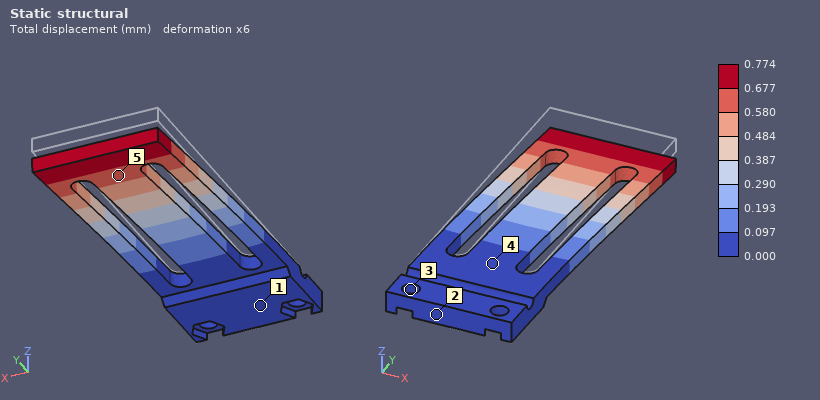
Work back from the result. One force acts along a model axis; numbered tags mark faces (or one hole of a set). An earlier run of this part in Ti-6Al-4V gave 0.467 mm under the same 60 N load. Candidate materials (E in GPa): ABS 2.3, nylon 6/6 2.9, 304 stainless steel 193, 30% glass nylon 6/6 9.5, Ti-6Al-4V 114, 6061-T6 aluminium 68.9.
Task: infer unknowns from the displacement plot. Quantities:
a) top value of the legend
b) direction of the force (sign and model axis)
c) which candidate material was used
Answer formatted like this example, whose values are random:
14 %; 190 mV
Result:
0.774 mm; -Z; 6061-T6 aluminium
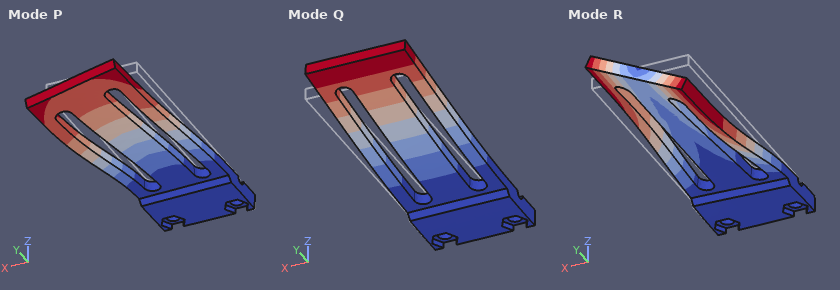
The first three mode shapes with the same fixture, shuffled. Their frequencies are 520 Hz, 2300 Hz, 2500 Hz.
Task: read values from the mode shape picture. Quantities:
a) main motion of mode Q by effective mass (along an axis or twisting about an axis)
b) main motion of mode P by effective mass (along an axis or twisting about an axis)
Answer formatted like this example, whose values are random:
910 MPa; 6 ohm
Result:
along Z; along X
